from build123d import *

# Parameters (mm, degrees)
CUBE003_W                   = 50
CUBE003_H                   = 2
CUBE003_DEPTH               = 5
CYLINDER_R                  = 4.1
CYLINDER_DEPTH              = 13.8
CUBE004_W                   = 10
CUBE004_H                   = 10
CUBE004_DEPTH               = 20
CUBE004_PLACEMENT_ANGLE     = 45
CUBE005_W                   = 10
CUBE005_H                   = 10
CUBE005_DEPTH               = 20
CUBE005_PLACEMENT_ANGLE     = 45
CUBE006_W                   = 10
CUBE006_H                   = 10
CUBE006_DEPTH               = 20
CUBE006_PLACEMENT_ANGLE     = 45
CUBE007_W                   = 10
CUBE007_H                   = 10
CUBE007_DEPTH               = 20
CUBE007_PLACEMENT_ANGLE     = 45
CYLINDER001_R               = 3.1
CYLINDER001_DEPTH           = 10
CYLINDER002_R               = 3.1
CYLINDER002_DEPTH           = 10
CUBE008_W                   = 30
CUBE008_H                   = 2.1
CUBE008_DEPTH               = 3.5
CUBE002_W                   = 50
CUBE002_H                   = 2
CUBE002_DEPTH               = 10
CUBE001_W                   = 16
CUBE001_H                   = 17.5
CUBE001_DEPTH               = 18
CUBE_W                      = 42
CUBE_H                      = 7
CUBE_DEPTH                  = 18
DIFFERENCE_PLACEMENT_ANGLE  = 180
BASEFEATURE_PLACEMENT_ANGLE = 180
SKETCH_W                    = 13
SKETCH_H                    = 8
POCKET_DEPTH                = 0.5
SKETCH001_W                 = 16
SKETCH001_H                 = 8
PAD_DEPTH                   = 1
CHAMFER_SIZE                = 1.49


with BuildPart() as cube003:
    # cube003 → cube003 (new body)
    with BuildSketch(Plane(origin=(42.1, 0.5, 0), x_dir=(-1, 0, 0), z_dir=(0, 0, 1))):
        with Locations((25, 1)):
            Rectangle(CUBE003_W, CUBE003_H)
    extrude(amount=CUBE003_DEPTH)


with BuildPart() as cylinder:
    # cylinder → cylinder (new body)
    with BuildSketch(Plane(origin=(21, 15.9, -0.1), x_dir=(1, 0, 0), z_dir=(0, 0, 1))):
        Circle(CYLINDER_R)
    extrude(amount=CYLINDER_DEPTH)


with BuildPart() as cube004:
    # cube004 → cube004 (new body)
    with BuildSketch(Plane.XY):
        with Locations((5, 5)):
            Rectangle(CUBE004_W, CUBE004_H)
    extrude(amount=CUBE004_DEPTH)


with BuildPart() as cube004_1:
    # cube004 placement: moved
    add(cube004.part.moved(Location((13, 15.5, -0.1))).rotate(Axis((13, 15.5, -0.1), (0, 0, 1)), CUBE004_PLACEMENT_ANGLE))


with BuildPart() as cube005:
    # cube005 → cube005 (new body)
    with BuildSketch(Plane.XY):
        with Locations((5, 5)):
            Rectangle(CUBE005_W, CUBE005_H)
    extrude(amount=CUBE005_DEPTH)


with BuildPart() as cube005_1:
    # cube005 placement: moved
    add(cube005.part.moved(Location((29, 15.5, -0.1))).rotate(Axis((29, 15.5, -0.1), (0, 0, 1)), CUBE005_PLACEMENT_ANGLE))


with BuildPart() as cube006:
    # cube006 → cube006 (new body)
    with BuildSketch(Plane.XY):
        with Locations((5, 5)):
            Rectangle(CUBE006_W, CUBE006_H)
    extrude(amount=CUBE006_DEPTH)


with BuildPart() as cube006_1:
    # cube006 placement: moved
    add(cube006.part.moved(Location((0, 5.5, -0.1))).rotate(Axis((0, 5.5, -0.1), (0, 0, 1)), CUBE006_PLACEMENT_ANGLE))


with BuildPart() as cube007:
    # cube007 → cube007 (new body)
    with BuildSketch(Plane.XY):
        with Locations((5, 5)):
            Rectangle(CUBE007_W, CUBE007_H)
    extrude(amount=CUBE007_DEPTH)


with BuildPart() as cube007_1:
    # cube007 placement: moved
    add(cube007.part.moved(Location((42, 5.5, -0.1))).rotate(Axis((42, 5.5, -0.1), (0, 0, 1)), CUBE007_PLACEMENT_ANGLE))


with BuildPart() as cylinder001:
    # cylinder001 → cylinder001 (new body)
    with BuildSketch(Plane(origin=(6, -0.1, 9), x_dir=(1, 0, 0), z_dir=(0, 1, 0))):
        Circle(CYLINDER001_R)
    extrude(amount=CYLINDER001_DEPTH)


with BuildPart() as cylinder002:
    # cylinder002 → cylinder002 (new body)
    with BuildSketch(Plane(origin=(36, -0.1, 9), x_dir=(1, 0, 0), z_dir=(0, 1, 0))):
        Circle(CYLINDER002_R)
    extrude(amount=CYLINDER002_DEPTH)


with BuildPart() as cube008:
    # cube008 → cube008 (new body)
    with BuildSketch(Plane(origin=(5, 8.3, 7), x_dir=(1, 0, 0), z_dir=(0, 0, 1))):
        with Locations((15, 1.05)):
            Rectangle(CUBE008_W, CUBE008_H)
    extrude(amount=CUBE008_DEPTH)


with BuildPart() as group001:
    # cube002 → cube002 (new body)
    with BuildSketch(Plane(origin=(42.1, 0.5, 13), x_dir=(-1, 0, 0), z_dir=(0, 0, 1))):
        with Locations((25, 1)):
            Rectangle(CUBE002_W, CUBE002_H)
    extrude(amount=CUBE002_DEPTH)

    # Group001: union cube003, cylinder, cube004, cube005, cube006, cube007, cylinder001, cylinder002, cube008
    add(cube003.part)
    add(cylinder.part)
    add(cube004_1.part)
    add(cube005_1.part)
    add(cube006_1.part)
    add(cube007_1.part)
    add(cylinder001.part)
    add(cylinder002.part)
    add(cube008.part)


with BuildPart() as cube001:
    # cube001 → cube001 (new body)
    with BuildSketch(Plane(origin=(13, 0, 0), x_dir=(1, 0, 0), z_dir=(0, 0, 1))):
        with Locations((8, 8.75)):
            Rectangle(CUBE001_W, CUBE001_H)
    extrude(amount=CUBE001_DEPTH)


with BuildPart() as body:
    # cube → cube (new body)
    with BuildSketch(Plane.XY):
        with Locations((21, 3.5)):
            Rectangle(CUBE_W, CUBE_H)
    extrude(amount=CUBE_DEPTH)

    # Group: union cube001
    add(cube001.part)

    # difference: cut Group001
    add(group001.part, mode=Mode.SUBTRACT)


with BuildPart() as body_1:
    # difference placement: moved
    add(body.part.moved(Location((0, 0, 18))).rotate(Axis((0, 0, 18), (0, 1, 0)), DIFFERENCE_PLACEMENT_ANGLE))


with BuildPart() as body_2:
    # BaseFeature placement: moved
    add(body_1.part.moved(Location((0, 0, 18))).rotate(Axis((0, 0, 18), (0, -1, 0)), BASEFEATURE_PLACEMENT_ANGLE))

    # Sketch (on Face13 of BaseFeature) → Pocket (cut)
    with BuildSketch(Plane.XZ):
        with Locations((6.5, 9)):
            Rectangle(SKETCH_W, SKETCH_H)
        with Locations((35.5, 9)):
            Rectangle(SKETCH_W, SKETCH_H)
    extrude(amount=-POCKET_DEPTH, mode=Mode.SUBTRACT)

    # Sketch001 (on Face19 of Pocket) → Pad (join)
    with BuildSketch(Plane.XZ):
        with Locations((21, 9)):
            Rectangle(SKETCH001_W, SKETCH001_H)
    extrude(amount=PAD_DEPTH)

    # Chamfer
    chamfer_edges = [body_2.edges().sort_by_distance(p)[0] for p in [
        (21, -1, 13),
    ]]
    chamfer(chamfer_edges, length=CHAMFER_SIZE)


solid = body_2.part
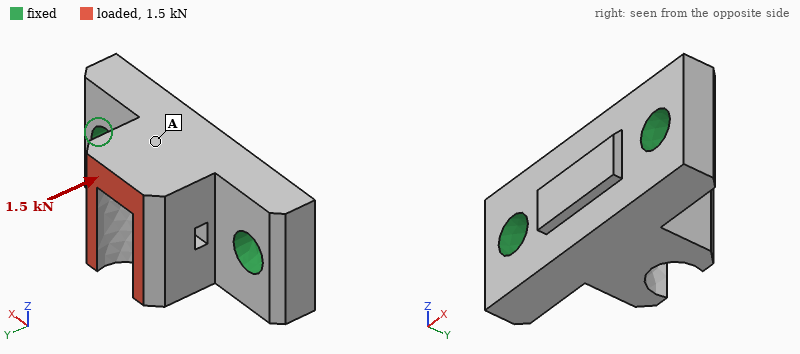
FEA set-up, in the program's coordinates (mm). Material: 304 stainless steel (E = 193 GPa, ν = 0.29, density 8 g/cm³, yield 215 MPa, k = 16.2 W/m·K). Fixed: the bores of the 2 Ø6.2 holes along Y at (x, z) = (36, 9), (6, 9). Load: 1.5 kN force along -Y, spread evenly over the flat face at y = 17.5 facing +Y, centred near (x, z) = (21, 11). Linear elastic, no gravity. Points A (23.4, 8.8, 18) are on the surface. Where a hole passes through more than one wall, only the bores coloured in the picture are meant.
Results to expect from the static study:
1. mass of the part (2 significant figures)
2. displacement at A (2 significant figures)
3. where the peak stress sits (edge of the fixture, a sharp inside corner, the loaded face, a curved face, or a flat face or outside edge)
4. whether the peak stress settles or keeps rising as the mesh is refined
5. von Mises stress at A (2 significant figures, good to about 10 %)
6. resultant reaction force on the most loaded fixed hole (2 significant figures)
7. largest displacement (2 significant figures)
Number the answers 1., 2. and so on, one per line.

1. 56 g
2. 2.5 µm
3. edge of the fixture
4. keeps rising
5. 7.5 MPa
6. 770 N
7. 3.3 µm
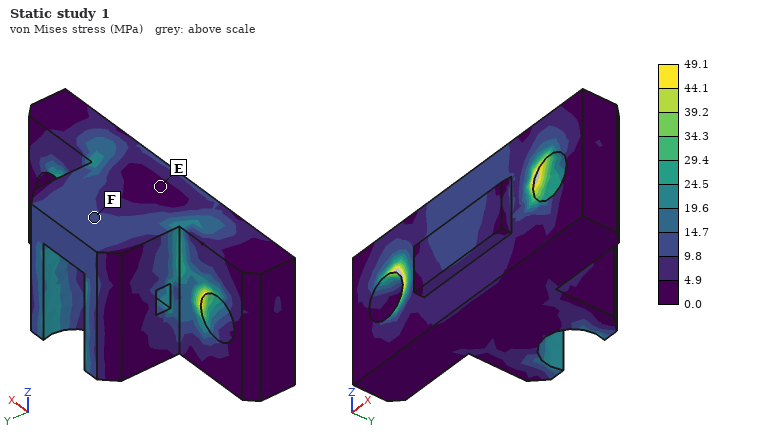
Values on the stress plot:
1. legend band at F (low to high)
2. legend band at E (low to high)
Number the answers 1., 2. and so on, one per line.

1. 9.8 to 14.7 MPa
2. 0.0 to 4.9 MPa
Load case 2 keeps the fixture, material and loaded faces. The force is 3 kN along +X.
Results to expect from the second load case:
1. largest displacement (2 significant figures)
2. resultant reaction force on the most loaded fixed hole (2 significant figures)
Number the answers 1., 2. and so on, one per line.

1. 12 µm
2. 2.4 kN
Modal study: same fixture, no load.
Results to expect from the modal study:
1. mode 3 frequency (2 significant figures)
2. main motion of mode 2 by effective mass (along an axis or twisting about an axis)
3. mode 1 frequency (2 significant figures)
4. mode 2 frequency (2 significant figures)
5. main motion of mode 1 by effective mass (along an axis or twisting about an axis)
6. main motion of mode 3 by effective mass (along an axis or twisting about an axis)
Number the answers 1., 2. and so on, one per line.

1. 33 kHz
2. along Y
3. 17 kHz
4. 27 kHz
5. along Z
6. along X
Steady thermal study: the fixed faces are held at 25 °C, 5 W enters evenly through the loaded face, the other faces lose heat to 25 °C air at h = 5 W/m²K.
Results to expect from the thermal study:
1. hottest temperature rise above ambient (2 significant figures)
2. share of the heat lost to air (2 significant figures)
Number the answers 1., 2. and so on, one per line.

1. 34 K
2. 3.1 %
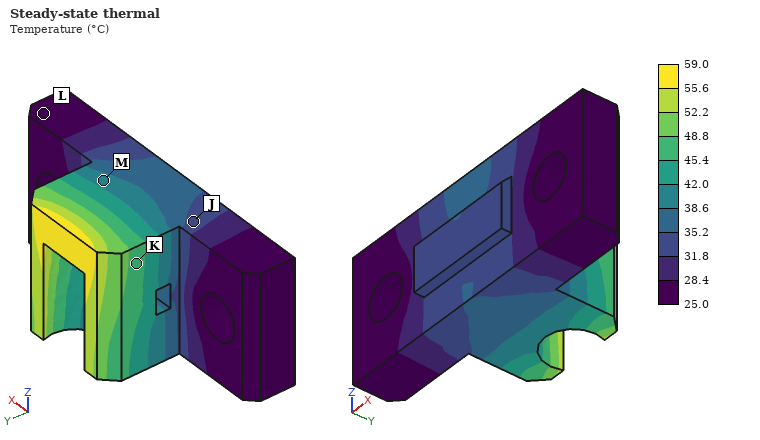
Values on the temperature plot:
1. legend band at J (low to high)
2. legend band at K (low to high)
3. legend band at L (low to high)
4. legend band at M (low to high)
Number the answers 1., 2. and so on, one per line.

1. 31.8 to 35.2 °C
2. 45.4 to 48.8 °C
3. 25.0 to 28.4 °C
4. 38.6 to 42.0 °C
